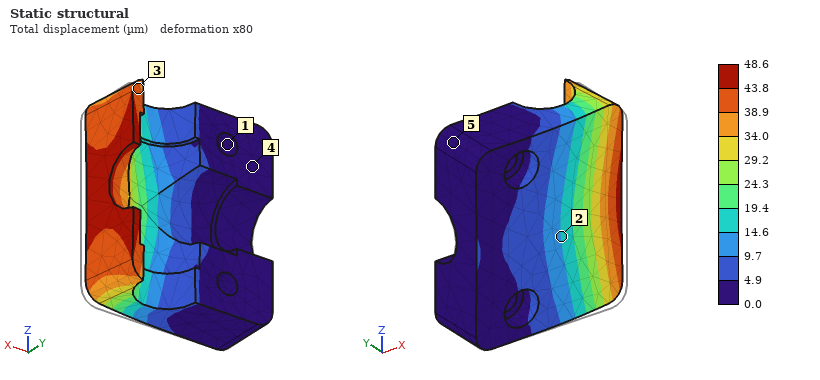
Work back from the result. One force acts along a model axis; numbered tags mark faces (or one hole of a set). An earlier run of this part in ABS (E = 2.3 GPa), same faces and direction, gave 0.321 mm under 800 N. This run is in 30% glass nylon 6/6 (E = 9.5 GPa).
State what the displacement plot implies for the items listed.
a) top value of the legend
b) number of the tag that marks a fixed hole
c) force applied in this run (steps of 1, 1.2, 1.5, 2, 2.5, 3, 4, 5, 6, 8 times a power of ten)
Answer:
48.6 µm
1
500 N
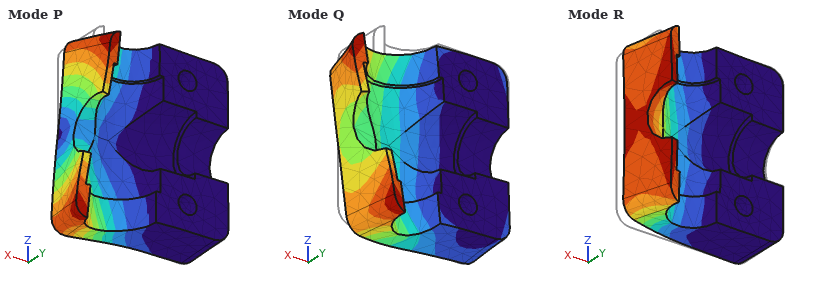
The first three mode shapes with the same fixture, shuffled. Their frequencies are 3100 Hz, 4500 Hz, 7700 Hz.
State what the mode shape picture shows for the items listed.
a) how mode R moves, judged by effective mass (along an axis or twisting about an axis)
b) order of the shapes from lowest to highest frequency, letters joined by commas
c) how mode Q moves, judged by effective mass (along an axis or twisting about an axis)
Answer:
along Y
R, P, Q
along Z
